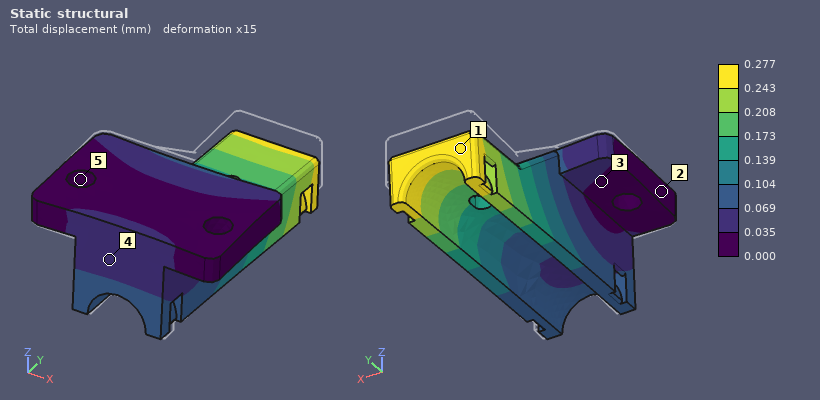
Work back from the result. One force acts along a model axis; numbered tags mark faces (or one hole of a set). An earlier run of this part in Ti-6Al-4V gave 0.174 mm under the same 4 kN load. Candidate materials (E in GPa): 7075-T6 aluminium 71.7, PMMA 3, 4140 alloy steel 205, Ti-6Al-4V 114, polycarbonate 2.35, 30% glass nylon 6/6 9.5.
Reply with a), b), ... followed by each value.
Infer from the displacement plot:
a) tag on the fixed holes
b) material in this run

a) 5
b) 7075-T6 aluminium
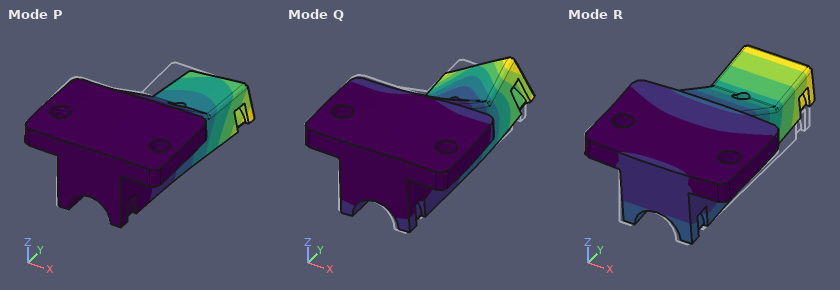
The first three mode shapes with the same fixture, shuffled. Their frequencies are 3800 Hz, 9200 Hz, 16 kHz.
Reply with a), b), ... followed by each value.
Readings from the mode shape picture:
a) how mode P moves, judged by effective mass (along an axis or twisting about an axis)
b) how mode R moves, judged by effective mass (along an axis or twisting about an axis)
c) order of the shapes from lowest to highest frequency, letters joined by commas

a) along X
b) along Z
c) R, P, Q
